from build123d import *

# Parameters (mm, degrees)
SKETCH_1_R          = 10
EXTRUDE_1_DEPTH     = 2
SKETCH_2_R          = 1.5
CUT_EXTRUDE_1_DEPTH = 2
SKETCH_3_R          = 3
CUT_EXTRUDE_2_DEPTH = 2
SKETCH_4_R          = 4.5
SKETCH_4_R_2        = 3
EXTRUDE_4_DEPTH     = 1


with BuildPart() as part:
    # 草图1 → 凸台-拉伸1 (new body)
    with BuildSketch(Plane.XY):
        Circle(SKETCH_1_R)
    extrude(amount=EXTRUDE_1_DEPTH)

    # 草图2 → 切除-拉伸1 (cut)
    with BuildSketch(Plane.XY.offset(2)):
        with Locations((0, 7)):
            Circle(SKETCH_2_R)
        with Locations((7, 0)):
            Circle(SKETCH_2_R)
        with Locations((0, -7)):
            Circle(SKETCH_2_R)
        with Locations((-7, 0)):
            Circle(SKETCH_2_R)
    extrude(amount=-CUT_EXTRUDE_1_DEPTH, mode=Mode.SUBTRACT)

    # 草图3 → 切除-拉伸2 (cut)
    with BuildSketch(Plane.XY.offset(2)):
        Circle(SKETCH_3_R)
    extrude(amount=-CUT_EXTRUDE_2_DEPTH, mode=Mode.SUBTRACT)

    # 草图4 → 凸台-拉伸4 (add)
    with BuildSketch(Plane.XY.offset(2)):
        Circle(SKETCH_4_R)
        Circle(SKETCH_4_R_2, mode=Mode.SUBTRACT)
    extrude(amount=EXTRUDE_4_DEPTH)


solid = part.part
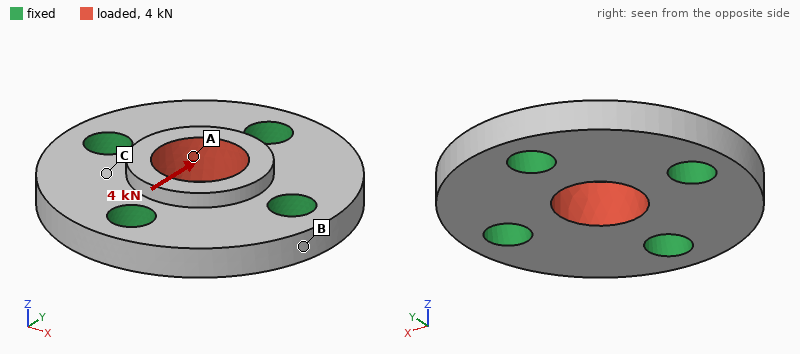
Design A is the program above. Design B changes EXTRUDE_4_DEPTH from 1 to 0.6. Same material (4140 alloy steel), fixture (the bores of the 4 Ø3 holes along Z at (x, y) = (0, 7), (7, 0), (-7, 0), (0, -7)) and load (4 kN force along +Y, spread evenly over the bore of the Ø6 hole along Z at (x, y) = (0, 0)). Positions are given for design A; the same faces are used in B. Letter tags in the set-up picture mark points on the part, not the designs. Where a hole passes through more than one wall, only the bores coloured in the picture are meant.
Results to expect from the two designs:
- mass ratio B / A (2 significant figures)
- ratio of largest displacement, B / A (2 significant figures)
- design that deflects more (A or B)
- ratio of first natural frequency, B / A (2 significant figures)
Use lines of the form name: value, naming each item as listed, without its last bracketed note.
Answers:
mass ratio B / A: 0.97
ratio of largest displacement, B / A: 0.86
design that deflects more: A
ratio of first natural frequency, B / A: 1.00
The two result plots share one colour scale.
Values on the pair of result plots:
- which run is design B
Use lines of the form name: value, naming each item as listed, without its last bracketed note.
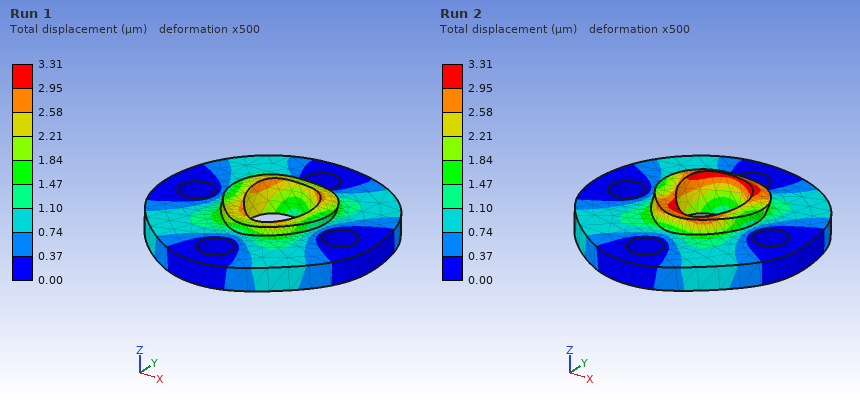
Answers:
which run is design B: Run 1
